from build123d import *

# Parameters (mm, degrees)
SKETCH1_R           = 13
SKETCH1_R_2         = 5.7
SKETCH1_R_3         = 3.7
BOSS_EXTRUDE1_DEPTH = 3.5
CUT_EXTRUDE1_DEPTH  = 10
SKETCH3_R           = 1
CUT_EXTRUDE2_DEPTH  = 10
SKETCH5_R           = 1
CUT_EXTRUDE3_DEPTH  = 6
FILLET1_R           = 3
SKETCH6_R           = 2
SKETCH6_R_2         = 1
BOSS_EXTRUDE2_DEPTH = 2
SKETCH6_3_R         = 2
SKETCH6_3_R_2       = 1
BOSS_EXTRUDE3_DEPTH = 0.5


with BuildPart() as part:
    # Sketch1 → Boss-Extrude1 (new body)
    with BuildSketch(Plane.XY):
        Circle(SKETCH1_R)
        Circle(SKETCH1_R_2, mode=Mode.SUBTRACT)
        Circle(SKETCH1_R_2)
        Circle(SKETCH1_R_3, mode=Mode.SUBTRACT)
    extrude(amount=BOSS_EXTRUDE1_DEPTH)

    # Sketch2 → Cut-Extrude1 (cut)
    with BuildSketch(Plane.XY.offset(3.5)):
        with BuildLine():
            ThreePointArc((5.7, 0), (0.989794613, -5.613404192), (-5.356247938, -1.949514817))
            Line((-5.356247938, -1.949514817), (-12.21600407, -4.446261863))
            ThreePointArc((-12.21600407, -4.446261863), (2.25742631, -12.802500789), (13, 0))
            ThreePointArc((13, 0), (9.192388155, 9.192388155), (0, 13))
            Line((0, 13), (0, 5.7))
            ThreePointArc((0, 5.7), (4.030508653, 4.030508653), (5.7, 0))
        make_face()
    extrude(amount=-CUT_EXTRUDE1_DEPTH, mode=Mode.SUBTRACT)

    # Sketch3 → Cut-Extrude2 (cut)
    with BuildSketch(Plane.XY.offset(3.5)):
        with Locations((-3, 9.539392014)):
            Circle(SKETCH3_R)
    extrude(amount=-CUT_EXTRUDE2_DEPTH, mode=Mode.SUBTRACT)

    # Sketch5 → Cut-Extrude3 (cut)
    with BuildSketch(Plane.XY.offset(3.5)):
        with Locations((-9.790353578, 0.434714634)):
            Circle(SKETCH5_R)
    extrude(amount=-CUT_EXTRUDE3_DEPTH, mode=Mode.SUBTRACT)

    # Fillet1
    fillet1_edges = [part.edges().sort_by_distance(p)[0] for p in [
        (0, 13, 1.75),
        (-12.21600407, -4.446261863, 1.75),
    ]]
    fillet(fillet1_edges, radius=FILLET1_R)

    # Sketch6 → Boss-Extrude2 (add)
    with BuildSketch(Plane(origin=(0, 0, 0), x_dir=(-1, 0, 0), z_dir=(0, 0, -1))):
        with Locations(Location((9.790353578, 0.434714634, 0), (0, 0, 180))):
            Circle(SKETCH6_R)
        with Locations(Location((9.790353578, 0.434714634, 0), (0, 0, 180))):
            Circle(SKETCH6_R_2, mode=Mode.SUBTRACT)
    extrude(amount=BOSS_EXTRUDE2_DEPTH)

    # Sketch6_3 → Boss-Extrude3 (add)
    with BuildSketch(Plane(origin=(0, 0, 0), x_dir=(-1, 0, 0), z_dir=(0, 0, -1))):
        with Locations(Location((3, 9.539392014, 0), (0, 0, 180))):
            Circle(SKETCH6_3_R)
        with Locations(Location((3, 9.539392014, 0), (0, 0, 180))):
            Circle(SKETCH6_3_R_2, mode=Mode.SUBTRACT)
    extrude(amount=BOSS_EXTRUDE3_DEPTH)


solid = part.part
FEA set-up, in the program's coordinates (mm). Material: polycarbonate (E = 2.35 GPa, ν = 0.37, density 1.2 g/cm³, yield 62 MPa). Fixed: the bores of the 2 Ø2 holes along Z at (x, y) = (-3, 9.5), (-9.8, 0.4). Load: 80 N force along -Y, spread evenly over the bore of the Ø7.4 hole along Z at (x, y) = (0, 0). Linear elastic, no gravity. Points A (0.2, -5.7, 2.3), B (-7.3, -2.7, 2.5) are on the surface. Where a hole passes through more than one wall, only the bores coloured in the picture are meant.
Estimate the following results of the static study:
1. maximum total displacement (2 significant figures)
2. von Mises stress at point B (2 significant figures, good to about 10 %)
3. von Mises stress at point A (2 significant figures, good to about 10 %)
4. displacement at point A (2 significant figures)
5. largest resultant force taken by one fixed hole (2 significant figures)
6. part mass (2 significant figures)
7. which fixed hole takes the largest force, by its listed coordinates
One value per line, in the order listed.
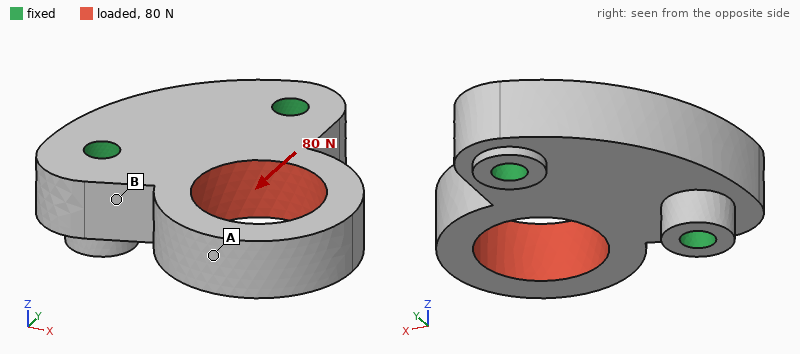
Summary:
0.17 mm
2.9 MPa
9.2 MPa
0.15 mm
75 N
0.78 g
(-3, 9.5)
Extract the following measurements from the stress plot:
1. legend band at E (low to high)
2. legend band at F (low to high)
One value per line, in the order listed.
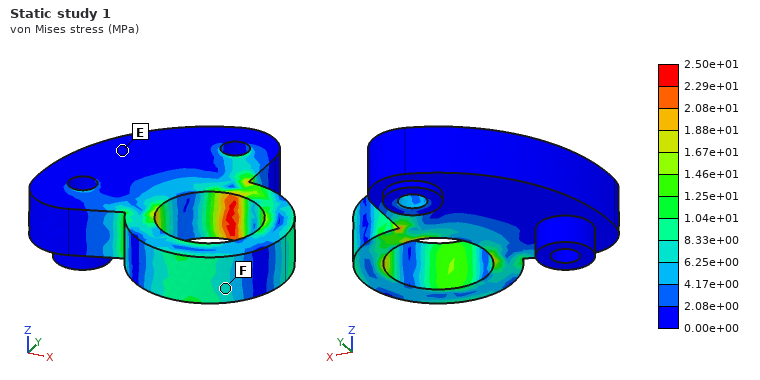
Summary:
0.00e+00 to 2.08e+00 MPa
6.25e+00 to 8.33e+00 MPa
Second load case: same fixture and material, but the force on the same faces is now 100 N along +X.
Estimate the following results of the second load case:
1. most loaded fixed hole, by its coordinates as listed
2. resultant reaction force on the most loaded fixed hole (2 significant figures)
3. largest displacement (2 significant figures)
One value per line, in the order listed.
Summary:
(-9.8, 0.4)
89 N
0.15 mm
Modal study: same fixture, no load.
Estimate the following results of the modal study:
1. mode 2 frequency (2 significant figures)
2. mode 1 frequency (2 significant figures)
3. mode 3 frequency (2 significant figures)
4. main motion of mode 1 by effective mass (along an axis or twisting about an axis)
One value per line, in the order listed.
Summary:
7000 Hz
4600 Hz
10 kHz
along Z
